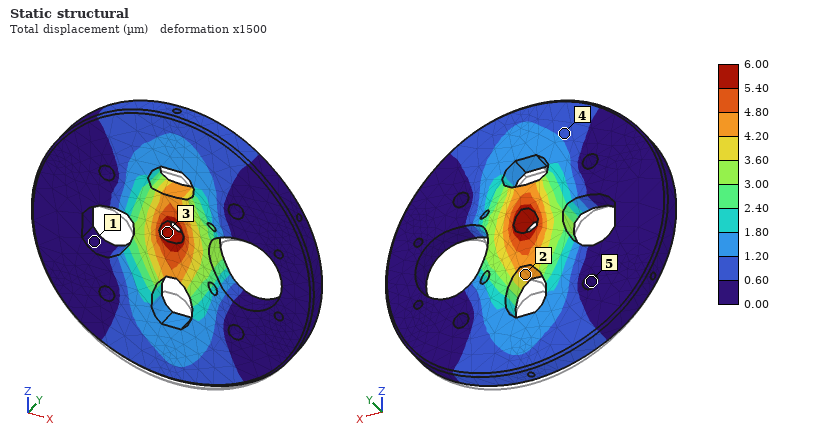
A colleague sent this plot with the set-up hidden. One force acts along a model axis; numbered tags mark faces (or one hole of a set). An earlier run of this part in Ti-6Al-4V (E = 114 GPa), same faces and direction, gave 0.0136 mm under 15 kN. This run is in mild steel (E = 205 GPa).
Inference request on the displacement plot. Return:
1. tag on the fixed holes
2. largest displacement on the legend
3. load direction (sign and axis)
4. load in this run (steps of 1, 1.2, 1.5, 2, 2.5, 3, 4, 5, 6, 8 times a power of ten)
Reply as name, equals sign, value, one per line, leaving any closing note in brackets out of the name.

tag on the fixed holes = 5
largest displacement on the legend = 6.00 µm
load direction = +Z
load in this run = 12 kN
